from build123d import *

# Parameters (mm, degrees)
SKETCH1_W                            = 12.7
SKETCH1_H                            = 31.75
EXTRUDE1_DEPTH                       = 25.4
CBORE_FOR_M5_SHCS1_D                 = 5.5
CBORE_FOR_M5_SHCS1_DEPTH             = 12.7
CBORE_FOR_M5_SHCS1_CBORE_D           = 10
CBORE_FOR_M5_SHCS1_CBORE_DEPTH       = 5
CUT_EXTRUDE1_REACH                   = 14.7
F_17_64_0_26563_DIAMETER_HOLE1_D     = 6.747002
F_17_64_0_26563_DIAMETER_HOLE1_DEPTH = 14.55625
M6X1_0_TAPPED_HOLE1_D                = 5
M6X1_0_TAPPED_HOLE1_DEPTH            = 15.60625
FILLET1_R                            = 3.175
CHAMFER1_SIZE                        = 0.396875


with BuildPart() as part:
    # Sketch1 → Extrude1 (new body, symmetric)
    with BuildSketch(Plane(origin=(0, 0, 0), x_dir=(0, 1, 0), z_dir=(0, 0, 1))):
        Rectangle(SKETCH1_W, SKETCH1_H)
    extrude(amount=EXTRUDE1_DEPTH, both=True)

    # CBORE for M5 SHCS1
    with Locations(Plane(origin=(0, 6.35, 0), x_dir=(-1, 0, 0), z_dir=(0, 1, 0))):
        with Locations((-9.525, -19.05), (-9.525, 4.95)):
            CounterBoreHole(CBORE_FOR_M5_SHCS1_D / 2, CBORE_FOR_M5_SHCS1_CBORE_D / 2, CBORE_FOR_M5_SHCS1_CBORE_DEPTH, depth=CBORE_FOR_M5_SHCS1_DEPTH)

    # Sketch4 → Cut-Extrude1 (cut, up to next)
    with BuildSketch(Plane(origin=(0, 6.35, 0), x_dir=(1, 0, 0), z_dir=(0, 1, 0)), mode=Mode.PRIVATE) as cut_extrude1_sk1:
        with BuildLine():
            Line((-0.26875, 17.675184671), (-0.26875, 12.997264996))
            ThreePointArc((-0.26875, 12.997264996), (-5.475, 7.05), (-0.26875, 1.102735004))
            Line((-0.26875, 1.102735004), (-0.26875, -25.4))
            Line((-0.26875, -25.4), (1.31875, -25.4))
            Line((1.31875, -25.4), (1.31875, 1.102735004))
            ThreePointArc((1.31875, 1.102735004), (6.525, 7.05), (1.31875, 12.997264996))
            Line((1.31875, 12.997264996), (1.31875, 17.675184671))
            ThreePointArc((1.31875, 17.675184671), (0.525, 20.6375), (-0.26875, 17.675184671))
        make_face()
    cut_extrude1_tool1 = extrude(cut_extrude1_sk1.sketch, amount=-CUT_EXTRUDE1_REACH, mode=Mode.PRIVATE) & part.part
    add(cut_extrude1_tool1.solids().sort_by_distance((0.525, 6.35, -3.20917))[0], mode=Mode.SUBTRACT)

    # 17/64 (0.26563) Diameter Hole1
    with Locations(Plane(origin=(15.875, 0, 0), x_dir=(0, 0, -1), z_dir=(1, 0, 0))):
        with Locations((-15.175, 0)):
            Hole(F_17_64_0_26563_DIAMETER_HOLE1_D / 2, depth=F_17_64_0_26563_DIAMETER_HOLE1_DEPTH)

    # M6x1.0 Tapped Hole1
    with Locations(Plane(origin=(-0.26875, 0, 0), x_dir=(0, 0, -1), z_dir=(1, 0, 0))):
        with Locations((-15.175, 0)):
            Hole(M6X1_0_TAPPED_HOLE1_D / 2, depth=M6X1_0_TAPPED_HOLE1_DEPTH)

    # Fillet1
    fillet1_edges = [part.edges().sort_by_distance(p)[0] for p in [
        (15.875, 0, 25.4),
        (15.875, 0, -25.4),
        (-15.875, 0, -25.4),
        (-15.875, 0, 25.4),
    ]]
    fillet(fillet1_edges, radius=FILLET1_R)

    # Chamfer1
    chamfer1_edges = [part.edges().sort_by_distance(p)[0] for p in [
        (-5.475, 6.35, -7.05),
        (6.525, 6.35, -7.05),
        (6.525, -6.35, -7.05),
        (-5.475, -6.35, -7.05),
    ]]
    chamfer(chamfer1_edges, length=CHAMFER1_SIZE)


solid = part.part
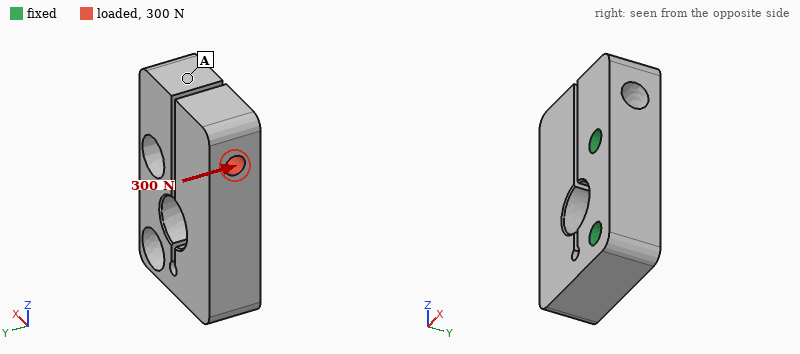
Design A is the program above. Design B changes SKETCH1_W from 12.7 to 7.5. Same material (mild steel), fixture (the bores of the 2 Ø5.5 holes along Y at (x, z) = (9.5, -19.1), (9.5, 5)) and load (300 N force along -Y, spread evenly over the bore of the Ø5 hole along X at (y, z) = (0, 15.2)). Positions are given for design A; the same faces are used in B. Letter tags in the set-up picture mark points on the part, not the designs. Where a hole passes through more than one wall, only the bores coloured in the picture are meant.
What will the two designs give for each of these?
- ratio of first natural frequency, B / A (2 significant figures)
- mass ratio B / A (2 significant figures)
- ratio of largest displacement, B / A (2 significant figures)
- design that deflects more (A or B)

1.0
0.57
3.3
B
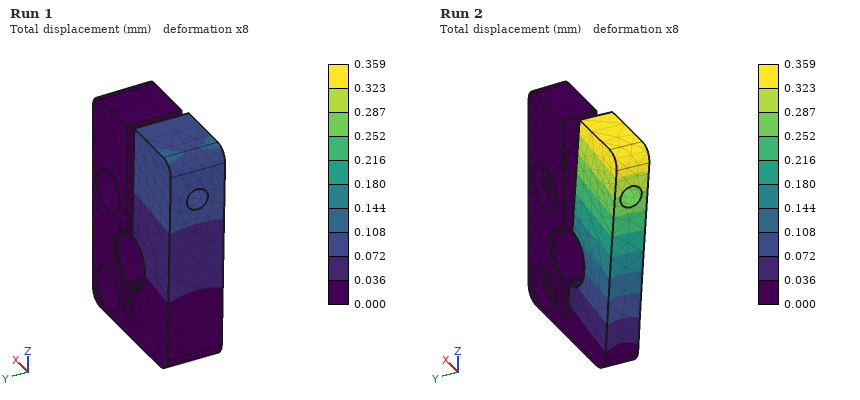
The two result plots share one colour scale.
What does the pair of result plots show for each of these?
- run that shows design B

Run 2
